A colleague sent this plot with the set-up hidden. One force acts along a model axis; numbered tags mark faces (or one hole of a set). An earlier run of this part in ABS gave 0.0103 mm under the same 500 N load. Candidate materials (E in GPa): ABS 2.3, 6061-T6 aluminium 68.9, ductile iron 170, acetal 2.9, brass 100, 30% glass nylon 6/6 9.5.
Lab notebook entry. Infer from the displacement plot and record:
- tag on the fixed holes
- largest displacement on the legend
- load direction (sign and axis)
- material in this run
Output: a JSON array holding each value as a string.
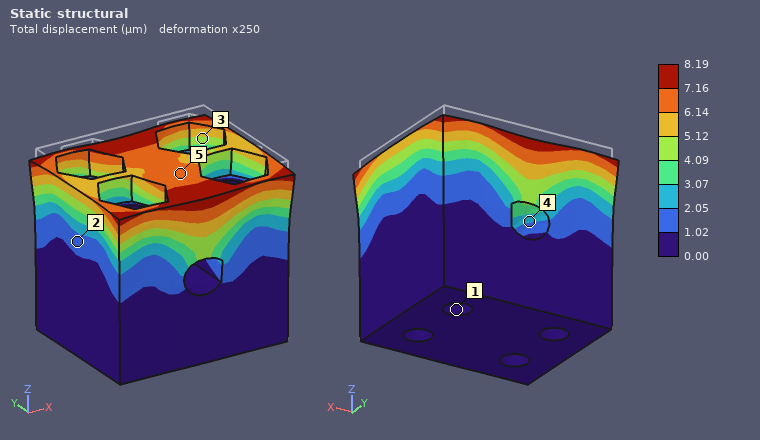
["1", "8.19 µm", "-Z", "acetal"]
